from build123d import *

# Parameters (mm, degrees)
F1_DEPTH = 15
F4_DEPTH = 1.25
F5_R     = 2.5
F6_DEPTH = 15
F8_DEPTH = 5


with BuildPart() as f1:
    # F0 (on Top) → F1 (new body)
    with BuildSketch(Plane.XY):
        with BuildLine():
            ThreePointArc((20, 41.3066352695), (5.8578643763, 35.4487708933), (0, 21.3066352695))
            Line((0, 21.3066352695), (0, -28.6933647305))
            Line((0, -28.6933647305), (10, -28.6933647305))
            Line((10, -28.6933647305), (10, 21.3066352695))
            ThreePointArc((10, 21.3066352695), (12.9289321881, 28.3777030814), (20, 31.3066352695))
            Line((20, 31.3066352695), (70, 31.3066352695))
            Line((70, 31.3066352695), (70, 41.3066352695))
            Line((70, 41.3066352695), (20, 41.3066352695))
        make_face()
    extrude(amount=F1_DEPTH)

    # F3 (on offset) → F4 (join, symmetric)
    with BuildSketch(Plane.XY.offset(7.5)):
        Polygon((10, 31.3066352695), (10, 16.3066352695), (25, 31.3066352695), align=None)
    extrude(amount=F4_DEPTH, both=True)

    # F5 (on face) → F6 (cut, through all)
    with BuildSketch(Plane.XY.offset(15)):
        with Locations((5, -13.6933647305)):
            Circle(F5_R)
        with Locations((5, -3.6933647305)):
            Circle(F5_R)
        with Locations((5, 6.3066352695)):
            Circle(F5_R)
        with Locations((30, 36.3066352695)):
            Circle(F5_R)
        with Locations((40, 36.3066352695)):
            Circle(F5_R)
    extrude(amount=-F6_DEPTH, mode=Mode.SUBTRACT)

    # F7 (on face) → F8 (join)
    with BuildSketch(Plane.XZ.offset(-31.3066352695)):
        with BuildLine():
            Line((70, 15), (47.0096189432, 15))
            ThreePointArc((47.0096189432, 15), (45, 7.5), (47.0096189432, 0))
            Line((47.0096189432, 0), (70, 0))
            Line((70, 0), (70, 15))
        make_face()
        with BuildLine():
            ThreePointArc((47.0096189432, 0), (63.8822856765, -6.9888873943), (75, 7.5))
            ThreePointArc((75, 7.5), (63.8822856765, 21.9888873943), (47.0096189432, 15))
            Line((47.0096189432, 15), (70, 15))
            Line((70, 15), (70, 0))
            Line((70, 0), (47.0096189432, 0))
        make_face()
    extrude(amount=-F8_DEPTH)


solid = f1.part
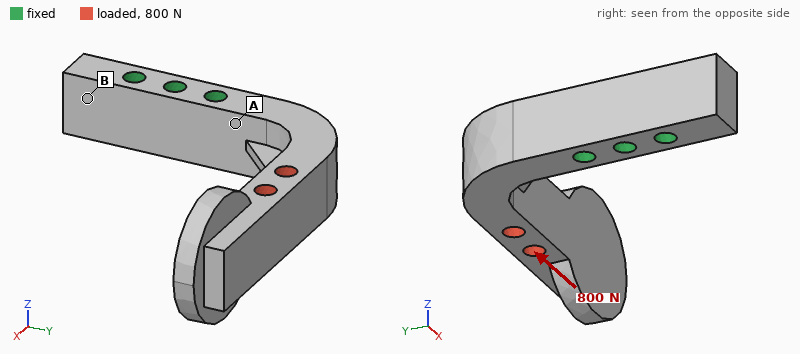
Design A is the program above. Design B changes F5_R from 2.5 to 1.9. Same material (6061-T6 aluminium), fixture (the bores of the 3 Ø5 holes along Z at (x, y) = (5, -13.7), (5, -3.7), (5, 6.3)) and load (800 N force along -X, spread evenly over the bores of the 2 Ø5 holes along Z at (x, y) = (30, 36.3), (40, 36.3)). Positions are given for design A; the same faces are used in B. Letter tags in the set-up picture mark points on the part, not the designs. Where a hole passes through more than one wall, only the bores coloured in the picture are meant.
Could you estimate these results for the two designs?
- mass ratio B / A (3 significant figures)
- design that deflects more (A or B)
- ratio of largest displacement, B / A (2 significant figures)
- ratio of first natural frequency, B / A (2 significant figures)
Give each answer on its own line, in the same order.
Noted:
1.03
B
1.1
0.97
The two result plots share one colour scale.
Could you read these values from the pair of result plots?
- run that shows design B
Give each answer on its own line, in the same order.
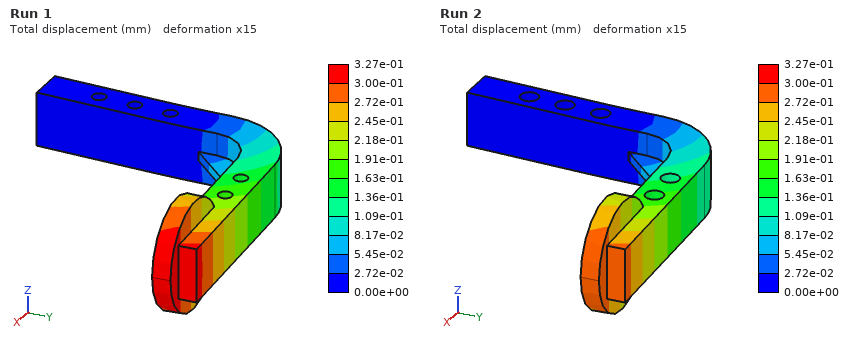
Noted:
Run 1
